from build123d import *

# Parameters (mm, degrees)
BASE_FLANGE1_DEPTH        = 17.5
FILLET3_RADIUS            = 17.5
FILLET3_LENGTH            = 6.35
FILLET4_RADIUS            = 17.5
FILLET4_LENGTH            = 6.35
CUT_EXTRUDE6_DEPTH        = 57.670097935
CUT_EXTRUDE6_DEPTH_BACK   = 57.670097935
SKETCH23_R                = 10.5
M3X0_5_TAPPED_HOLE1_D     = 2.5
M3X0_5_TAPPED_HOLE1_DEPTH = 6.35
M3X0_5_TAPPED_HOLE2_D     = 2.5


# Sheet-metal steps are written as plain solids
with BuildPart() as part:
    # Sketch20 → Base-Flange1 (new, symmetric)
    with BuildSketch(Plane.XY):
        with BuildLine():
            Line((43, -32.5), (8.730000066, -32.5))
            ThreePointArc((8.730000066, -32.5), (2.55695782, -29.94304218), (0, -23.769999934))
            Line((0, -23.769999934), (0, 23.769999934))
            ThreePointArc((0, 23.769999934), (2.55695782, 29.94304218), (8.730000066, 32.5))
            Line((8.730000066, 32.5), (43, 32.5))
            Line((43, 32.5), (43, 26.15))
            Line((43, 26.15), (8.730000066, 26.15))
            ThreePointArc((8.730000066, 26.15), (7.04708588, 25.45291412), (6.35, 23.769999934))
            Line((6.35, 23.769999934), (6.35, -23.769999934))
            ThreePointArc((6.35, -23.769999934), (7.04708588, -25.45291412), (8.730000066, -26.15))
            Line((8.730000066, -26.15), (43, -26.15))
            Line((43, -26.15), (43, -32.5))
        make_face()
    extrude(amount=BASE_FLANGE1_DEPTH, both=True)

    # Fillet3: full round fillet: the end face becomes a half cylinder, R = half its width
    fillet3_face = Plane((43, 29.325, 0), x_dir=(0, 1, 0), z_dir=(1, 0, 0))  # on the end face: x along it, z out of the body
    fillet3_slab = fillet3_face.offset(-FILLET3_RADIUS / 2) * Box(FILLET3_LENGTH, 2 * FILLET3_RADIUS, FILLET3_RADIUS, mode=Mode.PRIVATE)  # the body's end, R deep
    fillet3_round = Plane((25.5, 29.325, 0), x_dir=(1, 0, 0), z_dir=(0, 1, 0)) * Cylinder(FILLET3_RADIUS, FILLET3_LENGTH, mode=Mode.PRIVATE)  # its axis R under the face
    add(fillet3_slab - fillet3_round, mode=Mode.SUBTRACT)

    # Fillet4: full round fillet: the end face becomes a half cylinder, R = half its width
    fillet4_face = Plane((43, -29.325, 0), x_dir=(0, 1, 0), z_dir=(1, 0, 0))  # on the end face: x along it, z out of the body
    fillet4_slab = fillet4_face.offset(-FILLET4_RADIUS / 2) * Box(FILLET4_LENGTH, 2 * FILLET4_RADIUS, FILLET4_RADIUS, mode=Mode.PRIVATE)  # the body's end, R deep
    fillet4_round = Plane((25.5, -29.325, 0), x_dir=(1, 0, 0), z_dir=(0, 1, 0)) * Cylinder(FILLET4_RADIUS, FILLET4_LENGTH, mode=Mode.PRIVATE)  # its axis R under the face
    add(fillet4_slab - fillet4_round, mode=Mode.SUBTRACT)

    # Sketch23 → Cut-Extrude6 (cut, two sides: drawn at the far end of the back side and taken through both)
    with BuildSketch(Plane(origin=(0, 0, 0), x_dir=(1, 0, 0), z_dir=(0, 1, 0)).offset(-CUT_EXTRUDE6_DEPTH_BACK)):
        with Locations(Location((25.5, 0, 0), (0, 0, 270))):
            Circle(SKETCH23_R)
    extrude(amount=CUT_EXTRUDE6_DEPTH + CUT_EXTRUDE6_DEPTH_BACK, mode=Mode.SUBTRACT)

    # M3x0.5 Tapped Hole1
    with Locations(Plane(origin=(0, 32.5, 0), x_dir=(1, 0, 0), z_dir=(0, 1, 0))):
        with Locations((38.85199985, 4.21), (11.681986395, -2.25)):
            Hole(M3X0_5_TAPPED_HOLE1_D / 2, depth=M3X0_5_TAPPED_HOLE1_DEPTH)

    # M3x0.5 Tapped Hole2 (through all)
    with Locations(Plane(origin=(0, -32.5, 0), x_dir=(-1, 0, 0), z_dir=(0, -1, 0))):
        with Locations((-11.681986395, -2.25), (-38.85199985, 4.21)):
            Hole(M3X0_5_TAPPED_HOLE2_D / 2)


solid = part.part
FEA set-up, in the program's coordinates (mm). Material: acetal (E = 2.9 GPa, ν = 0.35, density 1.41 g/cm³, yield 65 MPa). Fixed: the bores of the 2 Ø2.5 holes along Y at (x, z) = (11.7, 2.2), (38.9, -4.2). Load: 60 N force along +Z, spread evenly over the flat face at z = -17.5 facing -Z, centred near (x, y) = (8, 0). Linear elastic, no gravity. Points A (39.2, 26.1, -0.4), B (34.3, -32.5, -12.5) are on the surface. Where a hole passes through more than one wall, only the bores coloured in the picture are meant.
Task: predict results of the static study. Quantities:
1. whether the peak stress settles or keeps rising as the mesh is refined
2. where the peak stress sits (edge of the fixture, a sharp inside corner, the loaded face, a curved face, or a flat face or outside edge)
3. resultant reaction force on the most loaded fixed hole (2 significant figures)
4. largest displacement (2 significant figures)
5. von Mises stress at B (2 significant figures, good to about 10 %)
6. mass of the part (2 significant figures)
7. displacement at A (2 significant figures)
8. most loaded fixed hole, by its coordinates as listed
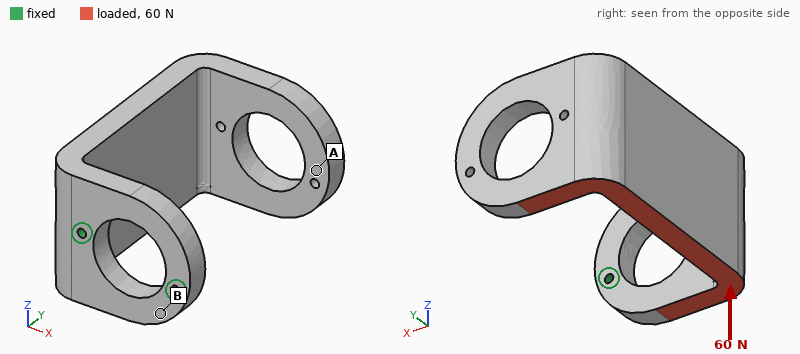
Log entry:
keeps rising
edge of the fixture
64 N
0.80 mm
2.9 MPa
33 g
0.72 mm
(11.7, 2.2)
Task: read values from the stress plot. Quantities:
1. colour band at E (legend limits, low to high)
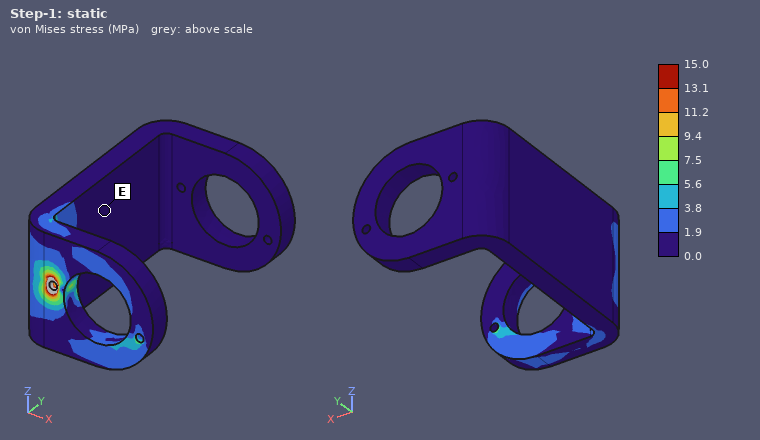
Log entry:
0.0 to 1.9 MPa
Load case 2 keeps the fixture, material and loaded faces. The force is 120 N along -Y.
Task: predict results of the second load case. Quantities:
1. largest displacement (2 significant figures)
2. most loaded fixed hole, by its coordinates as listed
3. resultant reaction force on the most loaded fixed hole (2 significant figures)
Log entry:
0.93 mm
(11.7, 2.2)
110 N
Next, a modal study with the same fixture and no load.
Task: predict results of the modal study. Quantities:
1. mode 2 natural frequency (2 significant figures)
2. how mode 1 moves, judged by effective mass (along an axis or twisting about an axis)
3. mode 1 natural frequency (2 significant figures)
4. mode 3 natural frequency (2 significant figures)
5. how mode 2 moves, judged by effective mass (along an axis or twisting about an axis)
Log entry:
280 Hz
along X
200 Hz
660 Hz
along Z
